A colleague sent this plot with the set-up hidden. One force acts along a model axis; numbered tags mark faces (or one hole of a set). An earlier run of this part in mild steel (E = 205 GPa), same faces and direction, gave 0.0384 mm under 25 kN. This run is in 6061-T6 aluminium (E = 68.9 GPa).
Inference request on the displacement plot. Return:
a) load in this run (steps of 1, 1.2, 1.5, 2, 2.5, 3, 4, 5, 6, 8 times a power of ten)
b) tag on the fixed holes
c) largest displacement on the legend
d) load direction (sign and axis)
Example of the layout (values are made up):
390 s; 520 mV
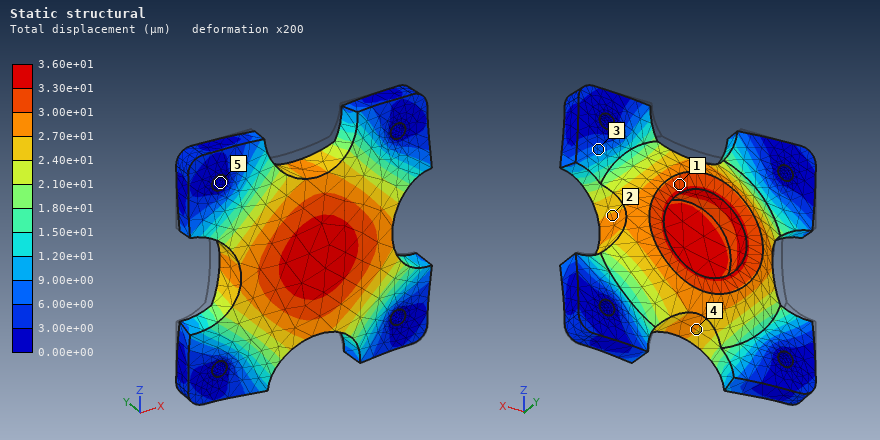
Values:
8 kN; 5; 3.60e+01 µm; -Y
